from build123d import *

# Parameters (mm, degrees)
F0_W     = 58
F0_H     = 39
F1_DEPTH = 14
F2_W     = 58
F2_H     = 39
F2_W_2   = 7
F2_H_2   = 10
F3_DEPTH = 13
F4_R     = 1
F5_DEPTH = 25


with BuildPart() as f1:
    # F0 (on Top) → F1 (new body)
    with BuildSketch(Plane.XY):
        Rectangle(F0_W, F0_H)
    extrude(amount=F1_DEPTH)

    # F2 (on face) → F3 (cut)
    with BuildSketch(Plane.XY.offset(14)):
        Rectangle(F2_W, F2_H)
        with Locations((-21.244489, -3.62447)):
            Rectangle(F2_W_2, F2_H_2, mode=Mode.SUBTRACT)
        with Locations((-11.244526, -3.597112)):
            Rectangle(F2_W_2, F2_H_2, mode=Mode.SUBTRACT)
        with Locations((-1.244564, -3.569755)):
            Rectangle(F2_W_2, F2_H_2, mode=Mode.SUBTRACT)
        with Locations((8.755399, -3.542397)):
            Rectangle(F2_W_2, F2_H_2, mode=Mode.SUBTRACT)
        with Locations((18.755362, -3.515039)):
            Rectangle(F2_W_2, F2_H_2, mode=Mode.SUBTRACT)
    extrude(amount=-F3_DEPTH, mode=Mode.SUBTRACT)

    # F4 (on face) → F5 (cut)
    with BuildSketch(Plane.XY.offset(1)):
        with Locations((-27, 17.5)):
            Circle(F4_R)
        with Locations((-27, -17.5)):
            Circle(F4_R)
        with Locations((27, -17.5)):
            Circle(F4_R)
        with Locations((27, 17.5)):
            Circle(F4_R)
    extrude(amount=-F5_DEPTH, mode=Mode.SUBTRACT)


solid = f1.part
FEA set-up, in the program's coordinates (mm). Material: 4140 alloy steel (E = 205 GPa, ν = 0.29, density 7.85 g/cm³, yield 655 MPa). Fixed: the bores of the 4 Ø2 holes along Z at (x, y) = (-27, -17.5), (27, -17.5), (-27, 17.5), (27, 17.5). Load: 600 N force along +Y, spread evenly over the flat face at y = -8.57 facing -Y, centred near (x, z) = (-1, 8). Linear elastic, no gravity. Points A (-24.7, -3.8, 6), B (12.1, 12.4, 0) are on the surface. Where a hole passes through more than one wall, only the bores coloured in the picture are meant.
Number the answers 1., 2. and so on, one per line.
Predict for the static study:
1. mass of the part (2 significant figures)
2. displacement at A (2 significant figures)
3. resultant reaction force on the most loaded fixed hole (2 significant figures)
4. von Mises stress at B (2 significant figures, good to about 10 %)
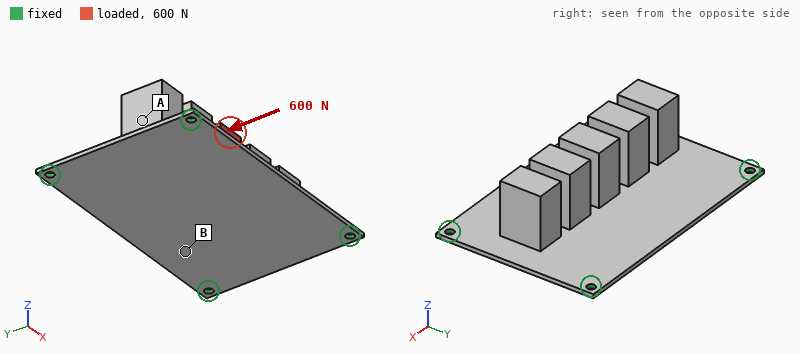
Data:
1. 53 g
2. 0.049 mm
3. 220 N
4. 58 MPa
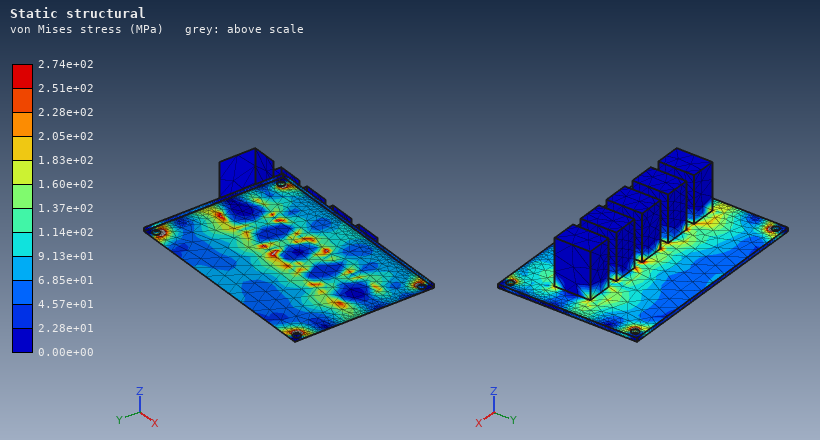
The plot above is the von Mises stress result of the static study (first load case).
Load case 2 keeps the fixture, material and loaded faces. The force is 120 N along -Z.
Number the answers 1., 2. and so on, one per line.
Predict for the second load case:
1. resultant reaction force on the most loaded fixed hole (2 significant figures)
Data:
1. 55 N
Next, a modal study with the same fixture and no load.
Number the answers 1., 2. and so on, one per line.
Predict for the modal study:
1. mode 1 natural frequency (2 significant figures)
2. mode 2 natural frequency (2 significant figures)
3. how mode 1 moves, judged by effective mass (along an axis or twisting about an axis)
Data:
1. 800 Hz
2. 1800 Hz
3. along Z
